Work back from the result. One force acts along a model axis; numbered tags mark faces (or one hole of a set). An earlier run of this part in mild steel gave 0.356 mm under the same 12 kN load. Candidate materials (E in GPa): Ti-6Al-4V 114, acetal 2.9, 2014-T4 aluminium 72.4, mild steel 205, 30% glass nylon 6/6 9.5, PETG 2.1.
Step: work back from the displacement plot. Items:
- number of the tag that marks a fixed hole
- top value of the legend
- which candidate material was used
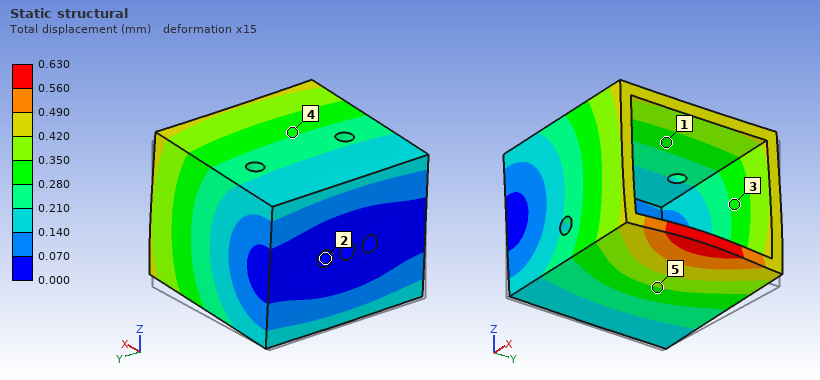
2
0.630 mm
Ti-6Al-4V
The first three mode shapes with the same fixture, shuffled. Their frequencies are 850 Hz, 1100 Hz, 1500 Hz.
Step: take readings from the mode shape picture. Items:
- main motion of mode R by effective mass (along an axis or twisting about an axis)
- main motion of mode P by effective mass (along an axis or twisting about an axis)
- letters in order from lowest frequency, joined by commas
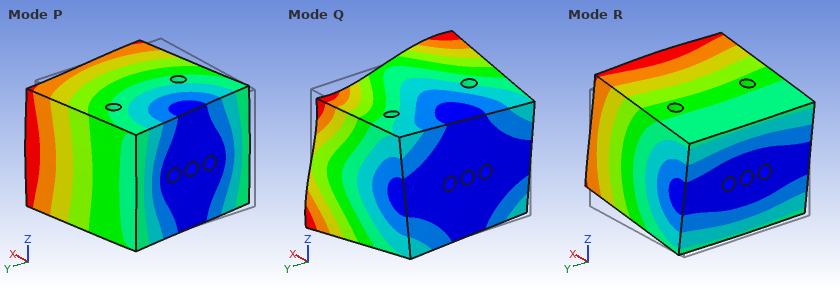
along Z
along Y
R, P, Q
